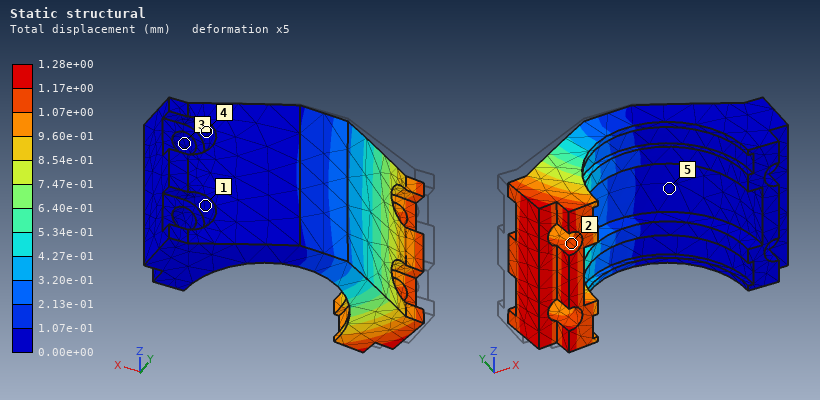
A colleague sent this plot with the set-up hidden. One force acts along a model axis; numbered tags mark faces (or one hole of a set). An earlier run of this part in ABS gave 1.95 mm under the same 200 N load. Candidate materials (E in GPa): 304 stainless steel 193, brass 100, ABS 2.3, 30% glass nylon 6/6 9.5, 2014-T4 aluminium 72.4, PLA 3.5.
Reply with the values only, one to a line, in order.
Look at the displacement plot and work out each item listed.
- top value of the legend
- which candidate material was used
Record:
1.28e+00 mm
PLA
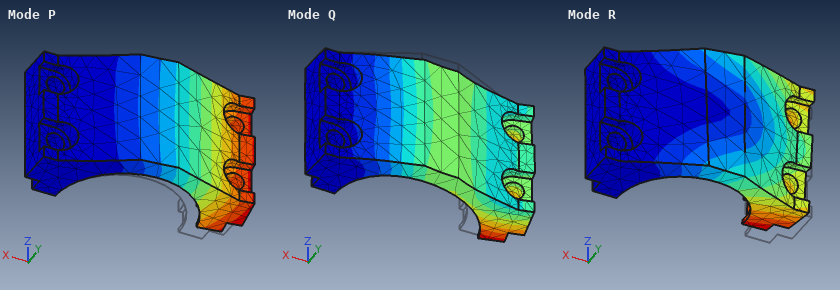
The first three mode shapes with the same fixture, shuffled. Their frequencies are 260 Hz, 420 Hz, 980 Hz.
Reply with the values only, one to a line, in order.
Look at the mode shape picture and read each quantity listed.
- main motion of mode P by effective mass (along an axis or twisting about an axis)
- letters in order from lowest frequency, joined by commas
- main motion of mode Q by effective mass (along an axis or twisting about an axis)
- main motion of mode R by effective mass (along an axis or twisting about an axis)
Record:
along Y
P, R, Q
along X
along Z
